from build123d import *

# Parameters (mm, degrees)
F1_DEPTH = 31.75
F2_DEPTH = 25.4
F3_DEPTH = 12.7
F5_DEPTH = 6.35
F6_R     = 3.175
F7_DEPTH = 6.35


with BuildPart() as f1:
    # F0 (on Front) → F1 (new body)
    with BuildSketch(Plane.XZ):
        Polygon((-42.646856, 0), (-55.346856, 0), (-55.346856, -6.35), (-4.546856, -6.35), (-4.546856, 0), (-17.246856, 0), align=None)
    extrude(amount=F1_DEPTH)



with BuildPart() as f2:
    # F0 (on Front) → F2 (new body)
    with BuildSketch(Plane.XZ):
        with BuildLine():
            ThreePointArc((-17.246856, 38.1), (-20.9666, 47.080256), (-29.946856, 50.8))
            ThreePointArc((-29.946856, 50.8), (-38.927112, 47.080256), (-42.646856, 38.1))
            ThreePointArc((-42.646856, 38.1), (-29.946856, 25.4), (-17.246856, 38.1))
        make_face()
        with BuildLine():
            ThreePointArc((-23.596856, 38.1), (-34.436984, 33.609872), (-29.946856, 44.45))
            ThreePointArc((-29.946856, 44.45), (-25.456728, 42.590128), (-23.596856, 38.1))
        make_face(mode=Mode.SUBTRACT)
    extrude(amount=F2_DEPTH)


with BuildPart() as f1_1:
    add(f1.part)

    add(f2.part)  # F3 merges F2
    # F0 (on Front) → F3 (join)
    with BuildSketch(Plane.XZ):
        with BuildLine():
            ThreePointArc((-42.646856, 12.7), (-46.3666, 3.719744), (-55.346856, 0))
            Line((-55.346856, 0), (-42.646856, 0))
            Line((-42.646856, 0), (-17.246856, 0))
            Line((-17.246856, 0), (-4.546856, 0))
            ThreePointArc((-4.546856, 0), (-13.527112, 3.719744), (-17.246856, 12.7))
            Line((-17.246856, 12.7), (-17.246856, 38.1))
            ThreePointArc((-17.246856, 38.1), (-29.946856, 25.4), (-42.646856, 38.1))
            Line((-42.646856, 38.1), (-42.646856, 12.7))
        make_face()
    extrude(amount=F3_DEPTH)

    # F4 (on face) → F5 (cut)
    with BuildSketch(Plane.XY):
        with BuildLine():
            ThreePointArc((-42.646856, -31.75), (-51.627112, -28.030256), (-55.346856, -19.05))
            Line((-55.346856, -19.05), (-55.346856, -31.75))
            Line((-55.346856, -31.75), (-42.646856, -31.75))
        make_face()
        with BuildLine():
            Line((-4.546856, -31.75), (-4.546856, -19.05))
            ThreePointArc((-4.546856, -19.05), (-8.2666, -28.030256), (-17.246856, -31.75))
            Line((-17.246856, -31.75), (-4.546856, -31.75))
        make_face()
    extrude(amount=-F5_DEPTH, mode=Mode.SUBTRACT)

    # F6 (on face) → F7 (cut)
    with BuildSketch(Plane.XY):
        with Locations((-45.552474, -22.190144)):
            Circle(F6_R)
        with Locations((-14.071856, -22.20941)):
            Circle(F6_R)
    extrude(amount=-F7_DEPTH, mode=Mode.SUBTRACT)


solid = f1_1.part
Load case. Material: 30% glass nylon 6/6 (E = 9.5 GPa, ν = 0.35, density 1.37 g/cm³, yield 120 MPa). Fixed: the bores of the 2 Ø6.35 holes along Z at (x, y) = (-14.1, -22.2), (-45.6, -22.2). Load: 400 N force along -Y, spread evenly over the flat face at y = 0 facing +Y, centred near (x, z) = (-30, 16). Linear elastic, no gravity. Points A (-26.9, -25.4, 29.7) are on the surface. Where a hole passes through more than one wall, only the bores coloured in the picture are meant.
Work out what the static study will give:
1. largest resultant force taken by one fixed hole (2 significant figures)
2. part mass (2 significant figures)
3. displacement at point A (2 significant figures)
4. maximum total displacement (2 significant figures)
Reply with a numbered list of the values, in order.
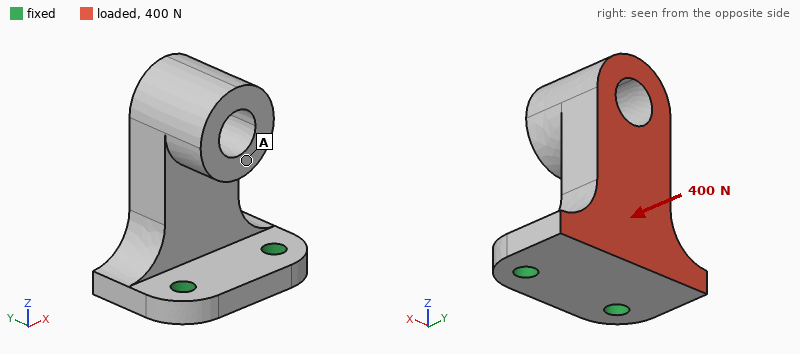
1. 210 N
2. 40 g
3. 0.37 mm
4. 0.61 mm
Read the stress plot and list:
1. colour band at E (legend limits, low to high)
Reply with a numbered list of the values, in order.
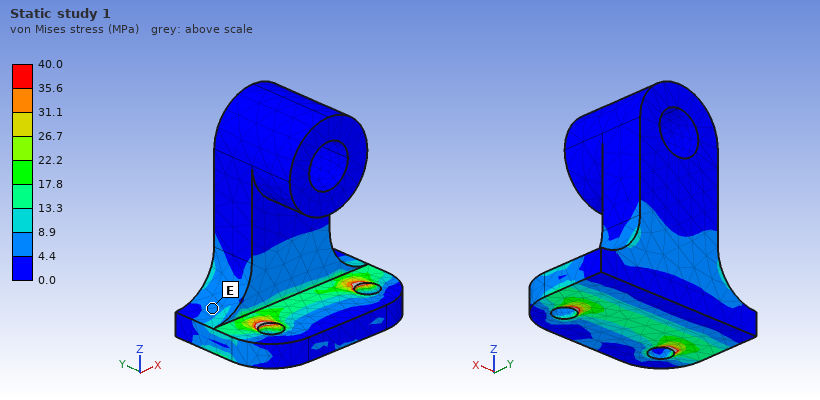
1. 4.4 to 8.9 MPa
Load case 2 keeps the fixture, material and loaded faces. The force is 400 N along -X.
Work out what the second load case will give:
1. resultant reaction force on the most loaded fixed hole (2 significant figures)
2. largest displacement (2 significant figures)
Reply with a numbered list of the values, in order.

1. 390 N
2. 96 µm
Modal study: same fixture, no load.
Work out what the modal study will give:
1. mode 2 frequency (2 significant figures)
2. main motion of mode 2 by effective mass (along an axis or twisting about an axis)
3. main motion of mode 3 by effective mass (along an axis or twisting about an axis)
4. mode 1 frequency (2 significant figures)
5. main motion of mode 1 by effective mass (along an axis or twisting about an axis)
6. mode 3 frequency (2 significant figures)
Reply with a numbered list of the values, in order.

1. 1800 Hz
2. along X
3. along Z
4. 770 Hz
5. along Y
6. 3400 Hz
